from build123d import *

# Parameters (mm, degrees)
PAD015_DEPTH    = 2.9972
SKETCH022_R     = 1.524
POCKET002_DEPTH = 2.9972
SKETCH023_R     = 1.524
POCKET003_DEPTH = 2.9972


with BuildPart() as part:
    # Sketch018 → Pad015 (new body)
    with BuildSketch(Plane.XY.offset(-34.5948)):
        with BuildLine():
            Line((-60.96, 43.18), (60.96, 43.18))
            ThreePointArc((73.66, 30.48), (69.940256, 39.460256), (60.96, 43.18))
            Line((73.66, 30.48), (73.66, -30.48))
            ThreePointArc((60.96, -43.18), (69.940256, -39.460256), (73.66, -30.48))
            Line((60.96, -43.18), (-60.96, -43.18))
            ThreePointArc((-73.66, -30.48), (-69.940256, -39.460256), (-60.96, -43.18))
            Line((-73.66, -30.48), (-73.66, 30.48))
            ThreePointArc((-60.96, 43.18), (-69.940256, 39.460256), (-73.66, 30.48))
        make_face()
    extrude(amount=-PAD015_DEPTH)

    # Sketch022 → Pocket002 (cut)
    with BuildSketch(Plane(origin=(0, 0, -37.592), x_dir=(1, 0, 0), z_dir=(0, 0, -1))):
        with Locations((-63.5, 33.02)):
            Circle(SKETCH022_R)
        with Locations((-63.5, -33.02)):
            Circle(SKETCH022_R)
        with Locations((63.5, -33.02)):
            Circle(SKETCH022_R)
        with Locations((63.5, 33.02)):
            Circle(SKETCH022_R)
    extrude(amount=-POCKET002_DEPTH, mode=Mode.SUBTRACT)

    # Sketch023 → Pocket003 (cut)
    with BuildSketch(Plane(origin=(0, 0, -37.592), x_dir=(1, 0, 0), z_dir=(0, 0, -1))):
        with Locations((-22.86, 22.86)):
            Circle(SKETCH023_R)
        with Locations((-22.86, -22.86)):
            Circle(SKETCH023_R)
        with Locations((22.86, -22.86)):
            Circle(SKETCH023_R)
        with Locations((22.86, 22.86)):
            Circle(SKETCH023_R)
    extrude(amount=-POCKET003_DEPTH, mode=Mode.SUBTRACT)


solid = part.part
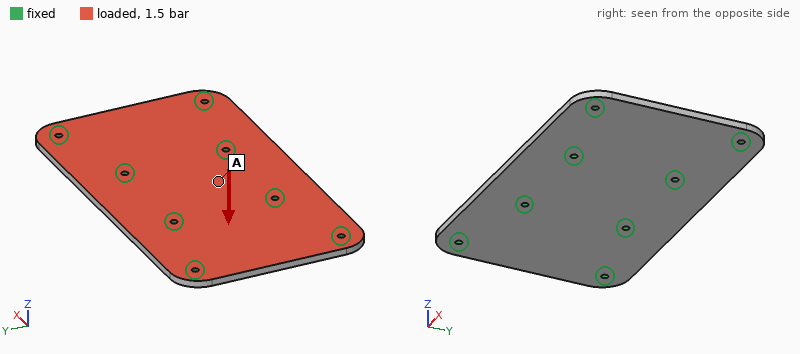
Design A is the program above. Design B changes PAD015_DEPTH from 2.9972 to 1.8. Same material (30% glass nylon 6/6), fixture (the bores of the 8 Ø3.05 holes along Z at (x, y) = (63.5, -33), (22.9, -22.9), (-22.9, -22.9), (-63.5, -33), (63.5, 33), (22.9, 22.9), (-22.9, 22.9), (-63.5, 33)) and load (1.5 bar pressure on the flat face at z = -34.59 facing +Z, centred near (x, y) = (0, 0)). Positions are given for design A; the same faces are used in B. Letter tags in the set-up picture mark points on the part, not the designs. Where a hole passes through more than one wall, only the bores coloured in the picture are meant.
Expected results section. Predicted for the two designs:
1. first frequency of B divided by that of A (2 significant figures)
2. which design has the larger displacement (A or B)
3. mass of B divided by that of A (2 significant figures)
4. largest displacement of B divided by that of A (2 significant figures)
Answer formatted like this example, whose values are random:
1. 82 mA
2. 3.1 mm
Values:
1. 0.63
2. B
3. 0.60
4. 4.3
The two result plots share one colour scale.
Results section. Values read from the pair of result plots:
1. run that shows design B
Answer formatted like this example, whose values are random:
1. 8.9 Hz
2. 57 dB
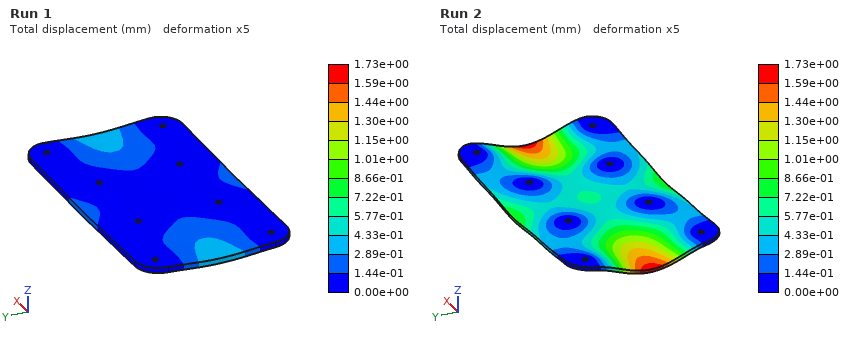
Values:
1. Run 2
